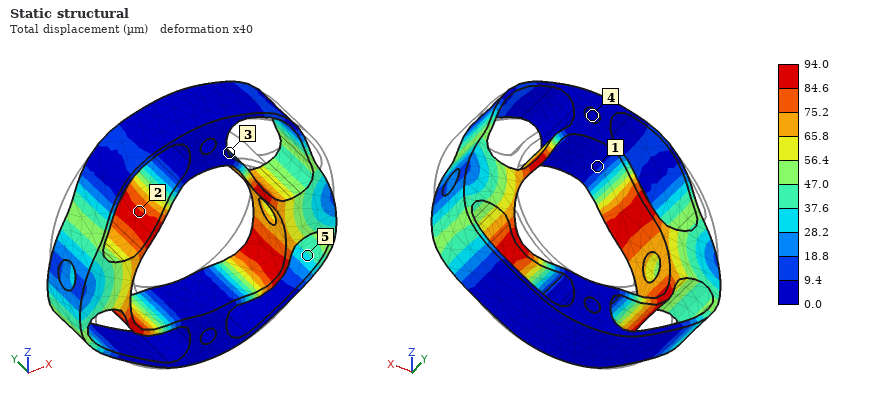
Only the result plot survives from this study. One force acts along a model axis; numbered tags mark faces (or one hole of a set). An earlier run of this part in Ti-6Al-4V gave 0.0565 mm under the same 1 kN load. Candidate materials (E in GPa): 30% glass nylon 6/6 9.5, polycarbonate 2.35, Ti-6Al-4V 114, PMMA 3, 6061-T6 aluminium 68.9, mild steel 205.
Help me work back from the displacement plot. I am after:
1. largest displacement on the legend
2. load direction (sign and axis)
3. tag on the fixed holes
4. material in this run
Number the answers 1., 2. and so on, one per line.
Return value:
1. 94.0 µm
2. -Z
3. 4
4. 6061-T6 aluminium
